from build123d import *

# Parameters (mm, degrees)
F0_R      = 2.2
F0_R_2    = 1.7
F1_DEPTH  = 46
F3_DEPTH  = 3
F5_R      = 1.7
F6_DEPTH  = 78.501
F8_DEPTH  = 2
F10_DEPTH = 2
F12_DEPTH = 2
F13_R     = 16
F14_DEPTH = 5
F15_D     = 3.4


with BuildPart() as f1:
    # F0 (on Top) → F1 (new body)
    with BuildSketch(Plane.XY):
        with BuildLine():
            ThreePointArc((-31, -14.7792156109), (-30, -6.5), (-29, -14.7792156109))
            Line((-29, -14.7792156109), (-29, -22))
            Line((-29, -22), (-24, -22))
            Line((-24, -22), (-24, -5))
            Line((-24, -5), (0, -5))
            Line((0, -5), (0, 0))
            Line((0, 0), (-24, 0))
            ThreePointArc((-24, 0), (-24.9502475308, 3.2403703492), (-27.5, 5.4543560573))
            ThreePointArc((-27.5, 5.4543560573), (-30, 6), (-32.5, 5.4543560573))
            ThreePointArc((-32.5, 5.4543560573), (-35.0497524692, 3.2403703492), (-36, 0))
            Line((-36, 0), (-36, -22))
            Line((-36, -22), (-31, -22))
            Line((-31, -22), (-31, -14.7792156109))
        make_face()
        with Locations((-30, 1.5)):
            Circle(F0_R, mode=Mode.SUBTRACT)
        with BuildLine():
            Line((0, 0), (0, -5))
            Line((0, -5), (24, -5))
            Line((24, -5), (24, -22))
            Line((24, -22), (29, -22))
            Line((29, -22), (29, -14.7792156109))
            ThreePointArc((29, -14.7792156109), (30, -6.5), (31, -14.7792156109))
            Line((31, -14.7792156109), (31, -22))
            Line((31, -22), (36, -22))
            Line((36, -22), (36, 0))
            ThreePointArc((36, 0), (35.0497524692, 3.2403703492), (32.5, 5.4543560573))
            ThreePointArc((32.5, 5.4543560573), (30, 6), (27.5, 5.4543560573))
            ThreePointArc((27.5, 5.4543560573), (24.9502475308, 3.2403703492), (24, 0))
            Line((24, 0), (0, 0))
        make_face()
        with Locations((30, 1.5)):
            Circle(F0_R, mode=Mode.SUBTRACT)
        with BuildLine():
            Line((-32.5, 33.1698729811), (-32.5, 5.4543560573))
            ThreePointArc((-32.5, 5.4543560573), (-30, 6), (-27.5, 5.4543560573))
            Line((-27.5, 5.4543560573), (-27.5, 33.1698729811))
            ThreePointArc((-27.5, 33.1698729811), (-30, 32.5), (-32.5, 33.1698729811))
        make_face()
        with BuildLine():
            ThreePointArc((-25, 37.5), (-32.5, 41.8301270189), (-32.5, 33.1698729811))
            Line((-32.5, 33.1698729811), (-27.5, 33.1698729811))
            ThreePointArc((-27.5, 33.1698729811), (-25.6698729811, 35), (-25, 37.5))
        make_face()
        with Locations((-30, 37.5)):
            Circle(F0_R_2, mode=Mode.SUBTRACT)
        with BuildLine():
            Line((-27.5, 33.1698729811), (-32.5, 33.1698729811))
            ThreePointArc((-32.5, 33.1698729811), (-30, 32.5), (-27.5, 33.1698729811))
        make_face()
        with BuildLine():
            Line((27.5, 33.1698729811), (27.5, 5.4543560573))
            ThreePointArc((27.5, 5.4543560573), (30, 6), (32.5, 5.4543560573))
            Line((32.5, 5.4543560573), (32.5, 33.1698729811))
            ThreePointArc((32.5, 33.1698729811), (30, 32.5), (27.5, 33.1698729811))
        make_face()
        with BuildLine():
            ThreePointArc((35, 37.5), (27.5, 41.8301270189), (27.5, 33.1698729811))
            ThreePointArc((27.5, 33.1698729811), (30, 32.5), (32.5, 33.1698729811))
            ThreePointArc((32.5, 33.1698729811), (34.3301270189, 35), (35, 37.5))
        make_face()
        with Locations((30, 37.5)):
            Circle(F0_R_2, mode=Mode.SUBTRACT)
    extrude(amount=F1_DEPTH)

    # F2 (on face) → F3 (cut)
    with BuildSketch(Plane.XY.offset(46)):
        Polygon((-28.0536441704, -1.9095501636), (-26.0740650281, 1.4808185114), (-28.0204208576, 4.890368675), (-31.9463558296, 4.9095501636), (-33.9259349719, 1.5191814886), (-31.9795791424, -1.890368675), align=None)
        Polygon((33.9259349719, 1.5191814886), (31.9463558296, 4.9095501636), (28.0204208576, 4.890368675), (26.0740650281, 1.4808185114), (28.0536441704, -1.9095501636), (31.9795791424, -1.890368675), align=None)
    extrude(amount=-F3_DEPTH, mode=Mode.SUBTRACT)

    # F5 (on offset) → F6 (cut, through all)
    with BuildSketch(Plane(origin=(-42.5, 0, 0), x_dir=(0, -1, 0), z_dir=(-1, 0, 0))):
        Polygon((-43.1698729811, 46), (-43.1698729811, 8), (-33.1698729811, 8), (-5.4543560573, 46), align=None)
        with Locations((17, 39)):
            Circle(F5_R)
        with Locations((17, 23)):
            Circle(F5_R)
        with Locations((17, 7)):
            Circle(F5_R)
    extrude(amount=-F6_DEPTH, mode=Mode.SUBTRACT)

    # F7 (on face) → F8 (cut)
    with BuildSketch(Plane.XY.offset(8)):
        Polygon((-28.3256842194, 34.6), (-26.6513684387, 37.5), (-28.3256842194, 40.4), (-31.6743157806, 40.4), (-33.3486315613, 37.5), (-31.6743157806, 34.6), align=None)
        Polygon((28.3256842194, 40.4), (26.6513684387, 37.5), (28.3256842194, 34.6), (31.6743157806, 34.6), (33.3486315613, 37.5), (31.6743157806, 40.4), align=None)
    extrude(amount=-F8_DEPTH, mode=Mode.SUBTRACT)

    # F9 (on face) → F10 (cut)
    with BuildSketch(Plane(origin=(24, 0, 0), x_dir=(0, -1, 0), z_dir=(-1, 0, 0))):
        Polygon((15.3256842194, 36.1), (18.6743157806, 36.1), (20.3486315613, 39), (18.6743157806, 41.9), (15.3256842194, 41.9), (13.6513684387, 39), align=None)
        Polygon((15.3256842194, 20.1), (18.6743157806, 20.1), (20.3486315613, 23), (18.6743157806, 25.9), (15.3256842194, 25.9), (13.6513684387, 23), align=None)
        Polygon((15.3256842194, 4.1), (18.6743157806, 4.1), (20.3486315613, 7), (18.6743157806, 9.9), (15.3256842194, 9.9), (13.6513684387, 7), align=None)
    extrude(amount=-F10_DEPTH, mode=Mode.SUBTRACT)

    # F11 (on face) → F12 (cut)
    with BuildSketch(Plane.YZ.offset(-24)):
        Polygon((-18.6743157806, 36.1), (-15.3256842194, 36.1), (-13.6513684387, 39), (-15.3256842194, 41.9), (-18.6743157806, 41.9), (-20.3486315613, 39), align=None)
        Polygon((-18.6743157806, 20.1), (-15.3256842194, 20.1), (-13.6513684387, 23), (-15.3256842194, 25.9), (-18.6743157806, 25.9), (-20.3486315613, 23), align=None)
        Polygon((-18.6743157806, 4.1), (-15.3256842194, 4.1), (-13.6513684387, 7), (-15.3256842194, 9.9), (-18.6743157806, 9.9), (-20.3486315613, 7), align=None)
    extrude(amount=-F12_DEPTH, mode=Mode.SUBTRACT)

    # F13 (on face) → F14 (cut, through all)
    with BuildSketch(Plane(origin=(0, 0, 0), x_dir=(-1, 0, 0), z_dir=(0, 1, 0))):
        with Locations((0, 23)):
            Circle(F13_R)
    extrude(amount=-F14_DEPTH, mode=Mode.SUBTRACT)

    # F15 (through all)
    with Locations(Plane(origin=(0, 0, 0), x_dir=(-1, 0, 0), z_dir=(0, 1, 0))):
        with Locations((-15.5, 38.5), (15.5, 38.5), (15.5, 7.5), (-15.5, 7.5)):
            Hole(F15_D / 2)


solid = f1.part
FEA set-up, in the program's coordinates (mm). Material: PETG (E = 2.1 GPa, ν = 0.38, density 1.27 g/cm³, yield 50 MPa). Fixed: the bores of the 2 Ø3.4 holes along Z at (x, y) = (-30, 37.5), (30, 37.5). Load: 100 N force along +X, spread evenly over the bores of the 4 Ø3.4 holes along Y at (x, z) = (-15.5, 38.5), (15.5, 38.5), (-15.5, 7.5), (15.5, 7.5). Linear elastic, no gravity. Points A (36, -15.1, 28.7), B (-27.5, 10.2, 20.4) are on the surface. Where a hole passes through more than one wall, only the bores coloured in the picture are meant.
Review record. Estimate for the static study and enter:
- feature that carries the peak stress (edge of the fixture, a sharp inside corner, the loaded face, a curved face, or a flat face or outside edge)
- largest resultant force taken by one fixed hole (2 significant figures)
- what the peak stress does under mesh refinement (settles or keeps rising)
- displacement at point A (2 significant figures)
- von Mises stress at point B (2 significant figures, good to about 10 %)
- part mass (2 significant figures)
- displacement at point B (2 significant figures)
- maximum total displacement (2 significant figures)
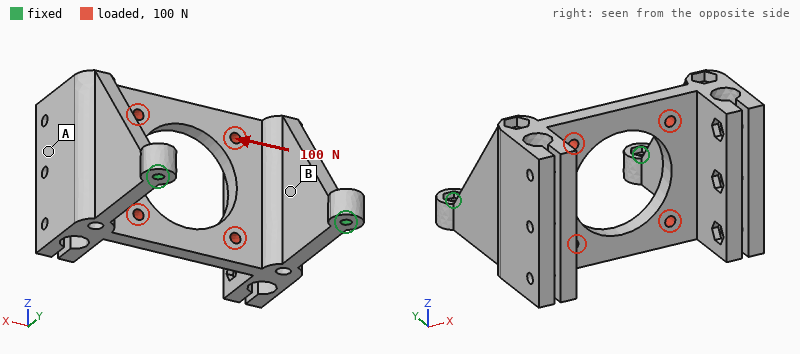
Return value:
edge of the fixture
68 N
keeps rising
0.99 mm
4.1 MPa
46 g
0.64 mm
1.1 mm
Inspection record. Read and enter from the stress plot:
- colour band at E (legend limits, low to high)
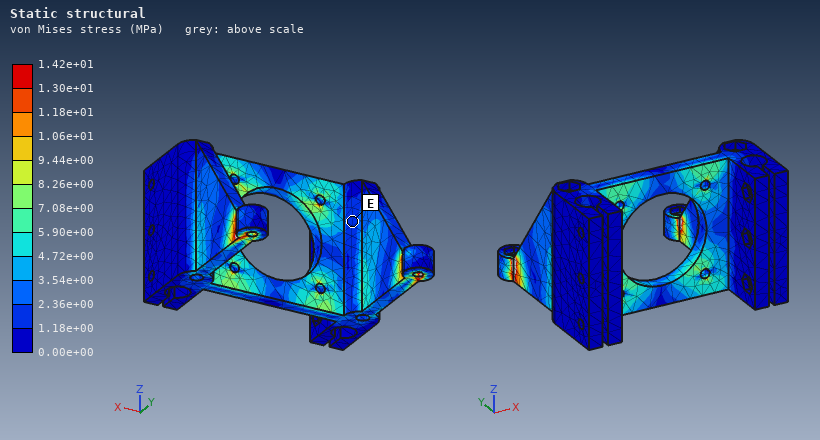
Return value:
1.18e+00 to 2.36e+00 MPa
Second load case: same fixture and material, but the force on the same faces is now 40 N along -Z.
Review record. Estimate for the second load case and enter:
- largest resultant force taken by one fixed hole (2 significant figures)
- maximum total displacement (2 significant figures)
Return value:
20 N
1.1 mm
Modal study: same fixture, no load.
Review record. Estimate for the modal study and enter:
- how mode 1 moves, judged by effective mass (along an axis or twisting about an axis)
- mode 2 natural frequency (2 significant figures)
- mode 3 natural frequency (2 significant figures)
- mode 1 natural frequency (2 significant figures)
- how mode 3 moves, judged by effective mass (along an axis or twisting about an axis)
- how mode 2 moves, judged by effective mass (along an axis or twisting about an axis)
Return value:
along Z
260 Hz
270 Hz
160 Hz
along X
along X
